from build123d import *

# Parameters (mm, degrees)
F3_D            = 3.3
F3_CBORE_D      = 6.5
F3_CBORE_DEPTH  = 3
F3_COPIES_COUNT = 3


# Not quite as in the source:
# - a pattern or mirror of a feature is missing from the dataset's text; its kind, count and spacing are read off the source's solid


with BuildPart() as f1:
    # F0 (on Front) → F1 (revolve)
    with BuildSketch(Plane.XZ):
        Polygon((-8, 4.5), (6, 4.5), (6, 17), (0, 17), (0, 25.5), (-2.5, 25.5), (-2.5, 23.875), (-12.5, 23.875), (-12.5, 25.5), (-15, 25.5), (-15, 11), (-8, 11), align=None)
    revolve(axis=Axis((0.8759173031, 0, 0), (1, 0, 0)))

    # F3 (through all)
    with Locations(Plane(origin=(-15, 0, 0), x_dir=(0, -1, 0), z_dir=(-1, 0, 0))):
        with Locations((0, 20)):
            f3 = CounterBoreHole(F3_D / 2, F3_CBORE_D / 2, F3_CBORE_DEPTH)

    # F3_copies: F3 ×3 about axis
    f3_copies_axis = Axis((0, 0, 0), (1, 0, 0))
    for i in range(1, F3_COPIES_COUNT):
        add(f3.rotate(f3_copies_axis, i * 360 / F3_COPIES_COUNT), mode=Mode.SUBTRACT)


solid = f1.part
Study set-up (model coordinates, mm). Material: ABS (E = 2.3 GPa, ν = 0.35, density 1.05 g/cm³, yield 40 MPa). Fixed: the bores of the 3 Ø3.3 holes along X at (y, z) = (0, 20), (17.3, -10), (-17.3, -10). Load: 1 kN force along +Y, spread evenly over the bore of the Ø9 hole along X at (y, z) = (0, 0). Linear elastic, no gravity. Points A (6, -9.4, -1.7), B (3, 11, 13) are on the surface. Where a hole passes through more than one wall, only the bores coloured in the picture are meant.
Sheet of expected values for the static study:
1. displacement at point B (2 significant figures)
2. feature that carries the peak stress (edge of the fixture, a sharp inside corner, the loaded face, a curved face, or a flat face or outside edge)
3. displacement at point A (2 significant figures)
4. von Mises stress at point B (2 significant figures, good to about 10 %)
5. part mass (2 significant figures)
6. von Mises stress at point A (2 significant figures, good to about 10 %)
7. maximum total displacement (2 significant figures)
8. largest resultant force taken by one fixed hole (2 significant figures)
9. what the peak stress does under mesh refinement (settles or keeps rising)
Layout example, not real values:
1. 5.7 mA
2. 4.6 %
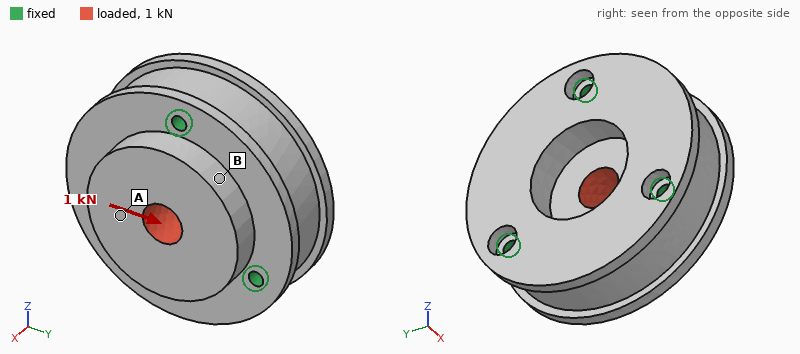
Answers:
1. 20 µm
2. edge of the fixture
3. 24 µm
4. 0.98 MPa
5. 31 g
6. 2.4 MPa
7. 32 µm
8. 370 N
9. keeps rising
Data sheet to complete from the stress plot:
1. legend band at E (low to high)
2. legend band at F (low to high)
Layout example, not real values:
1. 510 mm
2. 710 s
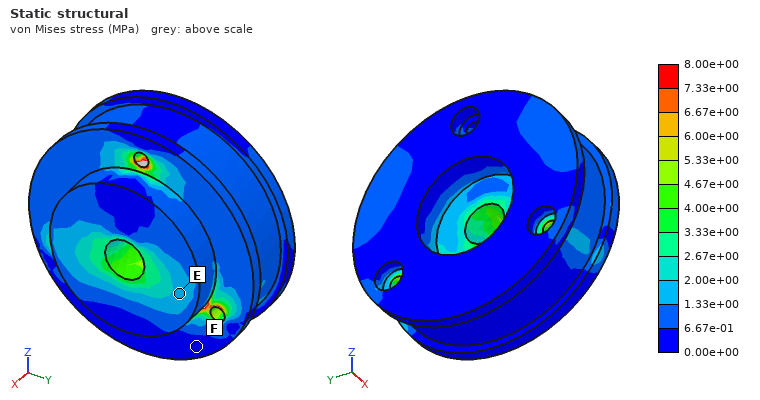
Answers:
1. 1.33e+00 to 2.00e+00 MPa
2. 0.00e+00 to 6.67e-01 MPa
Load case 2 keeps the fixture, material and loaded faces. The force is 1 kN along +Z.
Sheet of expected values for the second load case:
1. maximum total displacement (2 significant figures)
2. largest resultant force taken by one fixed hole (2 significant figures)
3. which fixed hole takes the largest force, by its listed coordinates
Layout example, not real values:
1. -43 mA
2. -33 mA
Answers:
1. 34 µm
2. 380 N
3. (0, 20)
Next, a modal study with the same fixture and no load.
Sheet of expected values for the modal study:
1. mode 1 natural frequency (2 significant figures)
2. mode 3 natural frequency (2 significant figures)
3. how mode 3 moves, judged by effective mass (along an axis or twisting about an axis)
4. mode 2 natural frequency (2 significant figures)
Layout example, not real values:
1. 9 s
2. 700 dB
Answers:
1. 6300 Hz
2. 7100 Hz
3. along X
4. 6300 Hz
